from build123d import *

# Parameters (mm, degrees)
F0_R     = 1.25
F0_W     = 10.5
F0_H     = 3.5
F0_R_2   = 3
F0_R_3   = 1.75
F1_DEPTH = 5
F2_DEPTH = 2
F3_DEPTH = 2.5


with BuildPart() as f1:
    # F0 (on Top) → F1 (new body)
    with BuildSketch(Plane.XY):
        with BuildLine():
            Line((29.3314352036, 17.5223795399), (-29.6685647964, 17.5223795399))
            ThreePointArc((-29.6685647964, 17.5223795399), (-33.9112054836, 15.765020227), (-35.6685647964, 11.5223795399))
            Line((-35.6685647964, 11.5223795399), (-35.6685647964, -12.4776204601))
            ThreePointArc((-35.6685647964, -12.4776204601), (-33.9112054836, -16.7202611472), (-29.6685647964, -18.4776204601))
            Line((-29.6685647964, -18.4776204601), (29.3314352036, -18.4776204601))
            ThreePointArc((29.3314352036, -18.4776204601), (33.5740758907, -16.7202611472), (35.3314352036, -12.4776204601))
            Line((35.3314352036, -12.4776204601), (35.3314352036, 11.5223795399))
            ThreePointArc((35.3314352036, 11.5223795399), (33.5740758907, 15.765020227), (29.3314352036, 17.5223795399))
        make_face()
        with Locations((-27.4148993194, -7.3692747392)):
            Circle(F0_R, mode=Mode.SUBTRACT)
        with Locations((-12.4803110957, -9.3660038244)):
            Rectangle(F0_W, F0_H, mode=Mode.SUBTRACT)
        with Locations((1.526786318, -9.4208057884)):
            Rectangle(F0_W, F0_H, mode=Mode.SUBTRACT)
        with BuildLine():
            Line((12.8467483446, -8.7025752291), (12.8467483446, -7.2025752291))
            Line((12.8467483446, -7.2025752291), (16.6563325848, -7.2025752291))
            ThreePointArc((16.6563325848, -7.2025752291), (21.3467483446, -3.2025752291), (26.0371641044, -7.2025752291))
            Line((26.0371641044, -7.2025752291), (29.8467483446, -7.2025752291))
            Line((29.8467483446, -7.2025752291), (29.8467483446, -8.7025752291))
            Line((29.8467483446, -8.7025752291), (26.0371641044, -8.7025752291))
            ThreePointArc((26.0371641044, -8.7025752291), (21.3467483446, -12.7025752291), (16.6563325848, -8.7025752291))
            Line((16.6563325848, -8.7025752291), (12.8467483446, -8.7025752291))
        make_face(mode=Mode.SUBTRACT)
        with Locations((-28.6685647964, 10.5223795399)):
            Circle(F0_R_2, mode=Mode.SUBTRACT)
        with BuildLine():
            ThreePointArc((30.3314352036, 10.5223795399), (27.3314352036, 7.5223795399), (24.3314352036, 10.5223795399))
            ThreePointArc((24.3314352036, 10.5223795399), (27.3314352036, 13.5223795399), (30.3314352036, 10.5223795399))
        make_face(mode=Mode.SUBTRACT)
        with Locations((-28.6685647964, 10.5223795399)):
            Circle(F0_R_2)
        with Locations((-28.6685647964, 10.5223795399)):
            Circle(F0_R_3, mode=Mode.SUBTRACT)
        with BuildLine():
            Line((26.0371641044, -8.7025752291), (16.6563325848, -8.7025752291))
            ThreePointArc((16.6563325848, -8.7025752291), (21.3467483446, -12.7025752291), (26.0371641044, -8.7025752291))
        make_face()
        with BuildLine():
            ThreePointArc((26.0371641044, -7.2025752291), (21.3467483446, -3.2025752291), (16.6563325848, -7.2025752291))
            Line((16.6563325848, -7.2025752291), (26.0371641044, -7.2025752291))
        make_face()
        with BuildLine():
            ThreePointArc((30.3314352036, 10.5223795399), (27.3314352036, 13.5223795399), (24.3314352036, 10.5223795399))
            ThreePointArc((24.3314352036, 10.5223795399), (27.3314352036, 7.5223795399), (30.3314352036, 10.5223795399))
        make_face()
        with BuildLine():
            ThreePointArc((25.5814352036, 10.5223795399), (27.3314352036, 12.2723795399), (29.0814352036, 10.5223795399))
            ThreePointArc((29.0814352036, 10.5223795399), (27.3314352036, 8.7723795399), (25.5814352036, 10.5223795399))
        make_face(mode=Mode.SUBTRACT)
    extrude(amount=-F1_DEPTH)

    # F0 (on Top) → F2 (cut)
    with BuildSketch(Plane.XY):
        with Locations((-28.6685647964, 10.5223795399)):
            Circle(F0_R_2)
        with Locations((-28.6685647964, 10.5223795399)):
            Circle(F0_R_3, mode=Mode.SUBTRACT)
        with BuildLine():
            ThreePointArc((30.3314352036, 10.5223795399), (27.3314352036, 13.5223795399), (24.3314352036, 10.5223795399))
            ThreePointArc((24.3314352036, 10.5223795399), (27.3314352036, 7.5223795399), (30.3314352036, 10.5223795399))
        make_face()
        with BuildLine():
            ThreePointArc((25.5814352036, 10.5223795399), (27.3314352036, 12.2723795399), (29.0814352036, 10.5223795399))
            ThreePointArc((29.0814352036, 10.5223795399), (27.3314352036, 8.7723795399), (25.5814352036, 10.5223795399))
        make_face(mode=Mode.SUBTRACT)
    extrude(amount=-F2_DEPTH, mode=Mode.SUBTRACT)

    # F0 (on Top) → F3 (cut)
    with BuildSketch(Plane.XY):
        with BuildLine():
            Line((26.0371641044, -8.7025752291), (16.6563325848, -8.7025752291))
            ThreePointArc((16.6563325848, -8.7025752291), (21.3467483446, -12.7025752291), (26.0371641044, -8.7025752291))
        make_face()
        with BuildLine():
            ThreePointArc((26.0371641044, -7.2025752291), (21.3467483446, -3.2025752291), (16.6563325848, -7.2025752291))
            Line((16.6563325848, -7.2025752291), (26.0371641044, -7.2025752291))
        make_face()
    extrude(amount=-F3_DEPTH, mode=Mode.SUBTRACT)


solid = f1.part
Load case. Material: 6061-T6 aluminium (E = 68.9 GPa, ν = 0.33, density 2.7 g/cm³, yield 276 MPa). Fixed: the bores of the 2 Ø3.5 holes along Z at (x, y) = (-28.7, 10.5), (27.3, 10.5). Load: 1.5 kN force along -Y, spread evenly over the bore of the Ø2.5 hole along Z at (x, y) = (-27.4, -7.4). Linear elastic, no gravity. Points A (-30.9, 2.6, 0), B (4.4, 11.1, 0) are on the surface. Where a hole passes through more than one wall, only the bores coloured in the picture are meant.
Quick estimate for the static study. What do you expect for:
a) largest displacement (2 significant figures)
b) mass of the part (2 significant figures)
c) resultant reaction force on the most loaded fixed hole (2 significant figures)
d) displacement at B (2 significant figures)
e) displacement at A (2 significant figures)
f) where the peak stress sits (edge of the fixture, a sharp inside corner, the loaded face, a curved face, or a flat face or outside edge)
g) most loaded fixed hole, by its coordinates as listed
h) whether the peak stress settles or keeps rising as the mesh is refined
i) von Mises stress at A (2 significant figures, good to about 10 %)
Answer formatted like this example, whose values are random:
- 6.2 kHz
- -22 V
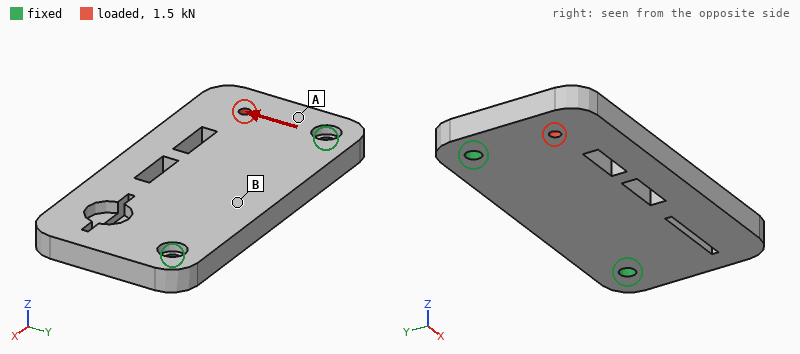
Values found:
- 22 µm
- 32 g
- 1.5 kN
- 3.5 µm
- 8.5 µm
- edge of the fixture
- (-28.7, 10.5)
- keeps rising
- 19 MPa
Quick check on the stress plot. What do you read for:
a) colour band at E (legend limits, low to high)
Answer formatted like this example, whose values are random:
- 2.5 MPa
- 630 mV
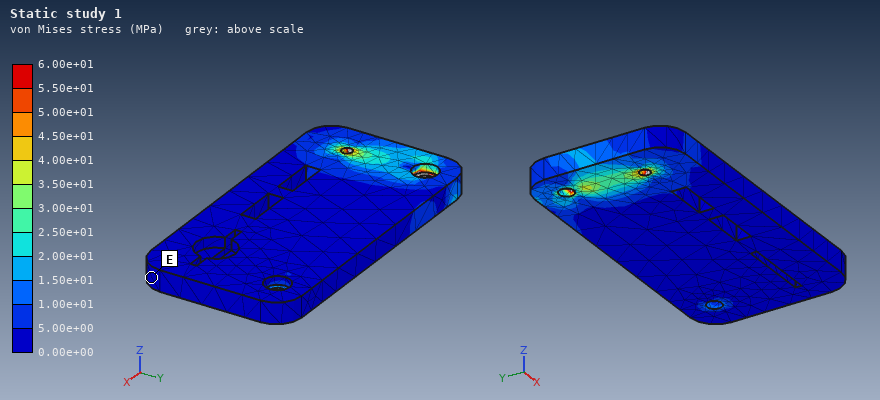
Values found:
- 0.00e+00 to 5.00e+00 MPa
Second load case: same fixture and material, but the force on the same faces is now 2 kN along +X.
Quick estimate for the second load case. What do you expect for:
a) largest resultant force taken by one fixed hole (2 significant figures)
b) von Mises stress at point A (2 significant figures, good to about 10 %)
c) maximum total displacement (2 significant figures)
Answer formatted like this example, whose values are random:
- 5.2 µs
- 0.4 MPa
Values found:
- 1.2 kN
- 9.1 MPa
- 17 µm
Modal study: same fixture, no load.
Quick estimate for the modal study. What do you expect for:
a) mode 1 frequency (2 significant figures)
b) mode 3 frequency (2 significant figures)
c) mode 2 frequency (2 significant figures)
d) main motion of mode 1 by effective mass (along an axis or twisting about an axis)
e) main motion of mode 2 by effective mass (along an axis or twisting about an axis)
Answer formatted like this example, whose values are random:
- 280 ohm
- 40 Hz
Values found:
- 2600 Hz
- 6500 Hz
- 5300 Hz
- along Z
- twisting about Y
